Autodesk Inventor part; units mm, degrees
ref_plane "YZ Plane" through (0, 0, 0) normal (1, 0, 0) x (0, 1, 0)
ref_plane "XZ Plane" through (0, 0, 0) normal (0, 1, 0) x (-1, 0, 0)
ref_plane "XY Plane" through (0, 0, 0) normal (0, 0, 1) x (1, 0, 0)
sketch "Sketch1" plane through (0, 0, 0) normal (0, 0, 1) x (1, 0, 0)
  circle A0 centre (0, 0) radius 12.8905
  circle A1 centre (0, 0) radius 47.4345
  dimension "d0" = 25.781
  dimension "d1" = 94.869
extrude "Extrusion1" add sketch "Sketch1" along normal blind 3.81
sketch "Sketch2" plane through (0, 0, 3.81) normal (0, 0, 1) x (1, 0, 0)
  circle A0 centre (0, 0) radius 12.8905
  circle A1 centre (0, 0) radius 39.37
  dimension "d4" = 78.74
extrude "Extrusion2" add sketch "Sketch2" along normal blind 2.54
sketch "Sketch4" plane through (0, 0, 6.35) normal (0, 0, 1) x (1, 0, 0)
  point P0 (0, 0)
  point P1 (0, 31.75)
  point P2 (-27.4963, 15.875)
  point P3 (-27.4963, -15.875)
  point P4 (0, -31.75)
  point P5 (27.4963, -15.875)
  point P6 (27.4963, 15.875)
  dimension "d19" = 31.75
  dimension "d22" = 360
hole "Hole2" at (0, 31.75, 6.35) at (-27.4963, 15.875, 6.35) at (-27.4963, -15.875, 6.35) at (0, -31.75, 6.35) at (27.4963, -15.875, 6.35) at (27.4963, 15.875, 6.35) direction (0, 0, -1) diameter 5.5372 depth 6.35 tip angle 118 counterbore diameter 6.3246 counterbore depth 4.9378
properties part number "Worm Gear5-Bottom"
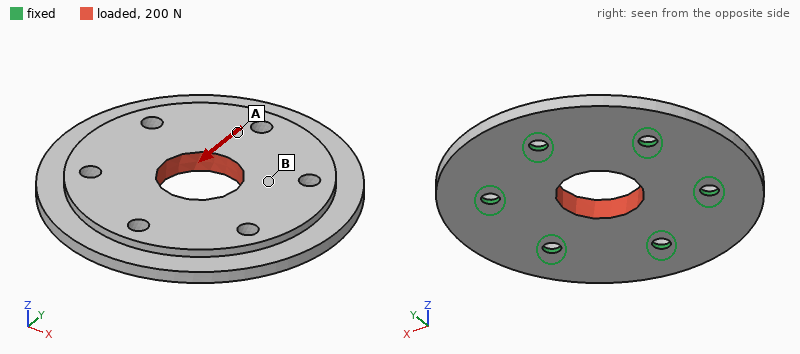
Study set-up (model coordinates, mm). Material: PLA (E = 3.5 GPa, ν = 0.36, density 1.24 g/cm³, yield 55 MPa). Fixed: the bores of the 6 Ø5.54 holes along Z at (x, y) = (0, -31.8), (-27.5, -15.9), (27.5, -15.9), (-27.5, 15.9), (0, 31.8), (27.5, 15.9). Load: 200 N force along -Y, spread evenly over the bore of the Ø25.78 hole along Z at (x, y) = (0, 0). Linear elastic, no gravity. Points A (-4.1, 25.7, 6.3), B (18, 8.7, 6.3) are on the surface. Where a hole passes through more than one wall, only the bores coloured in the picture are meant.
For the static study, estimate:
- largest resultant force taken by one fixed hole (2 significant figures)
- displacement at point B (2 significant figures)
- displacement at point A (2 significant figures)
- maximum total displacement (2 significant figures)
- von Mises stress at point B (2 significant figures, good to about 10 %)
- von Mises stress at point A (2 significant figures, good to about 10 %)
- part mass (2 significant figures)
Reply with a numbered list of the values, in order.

1. 41 N
2. 2.6 µm
3. 3.4 µm
4. 5.4 µm
5. 0.22 MPa
6. 0.40 MPa
7. 43 g
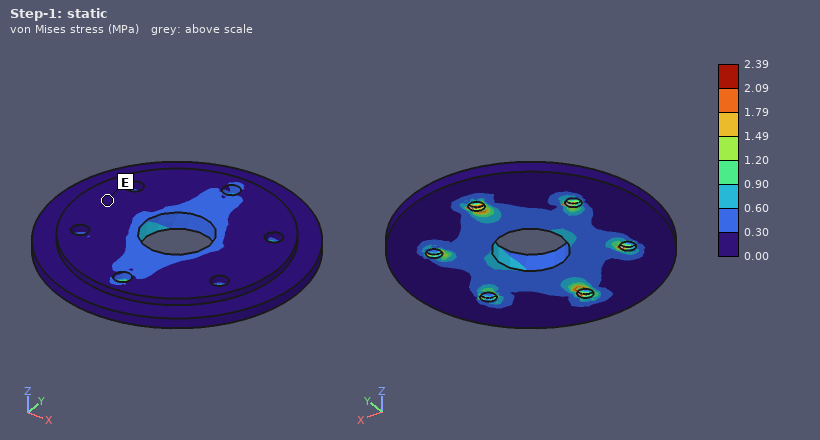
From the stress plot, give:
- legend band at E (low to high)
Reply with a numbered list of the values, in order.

1. 0.00 to 0.30 MPa
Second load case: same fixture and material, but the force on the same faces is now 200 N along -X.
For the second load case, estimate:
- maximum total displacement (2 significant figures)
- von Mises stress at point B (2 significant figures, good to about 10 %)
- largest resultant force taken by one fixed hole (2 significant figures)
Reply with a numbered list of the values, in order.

1. 5.6 µm
2. 0.37 MPa
3. 38 N
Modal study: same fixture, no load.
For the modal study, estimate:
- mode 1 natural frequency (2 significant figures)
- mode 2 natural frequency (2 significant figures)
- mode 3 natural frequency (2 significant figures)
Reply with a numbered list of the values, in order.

1. 3200 Hz
2. 3600 Hz
3. 3700 Hz
